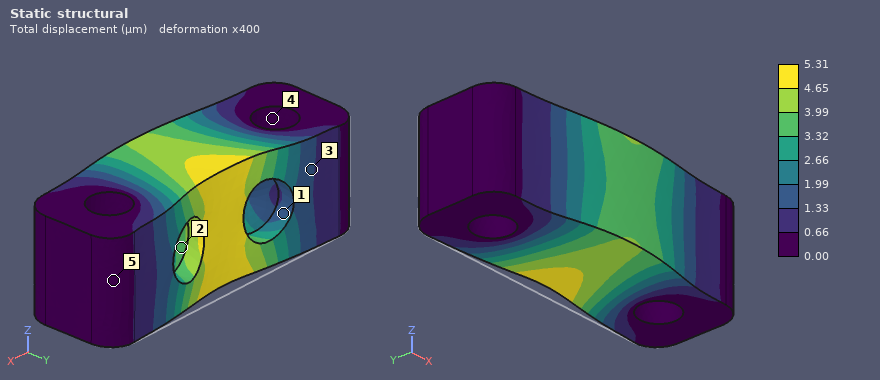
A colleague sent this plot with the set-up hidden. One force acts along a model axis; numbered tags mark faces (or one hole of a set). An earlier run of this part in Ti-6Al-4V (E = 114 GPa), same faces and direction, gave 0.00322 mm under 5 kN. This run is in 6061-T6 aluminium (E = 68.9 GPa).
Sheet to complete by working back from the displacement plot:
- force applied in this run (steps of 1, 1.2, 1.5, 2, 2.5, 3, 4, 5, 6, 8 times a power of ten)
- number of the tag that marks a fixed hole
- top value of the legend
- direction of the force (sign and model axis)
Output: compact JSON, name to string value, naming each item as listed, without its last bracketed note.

{"force applied in this run": "5 kN", "number of the tag that marks a fixed hole": "4", "top value of the legend": "5.31 µm", "direction of the force": "-Y"}
